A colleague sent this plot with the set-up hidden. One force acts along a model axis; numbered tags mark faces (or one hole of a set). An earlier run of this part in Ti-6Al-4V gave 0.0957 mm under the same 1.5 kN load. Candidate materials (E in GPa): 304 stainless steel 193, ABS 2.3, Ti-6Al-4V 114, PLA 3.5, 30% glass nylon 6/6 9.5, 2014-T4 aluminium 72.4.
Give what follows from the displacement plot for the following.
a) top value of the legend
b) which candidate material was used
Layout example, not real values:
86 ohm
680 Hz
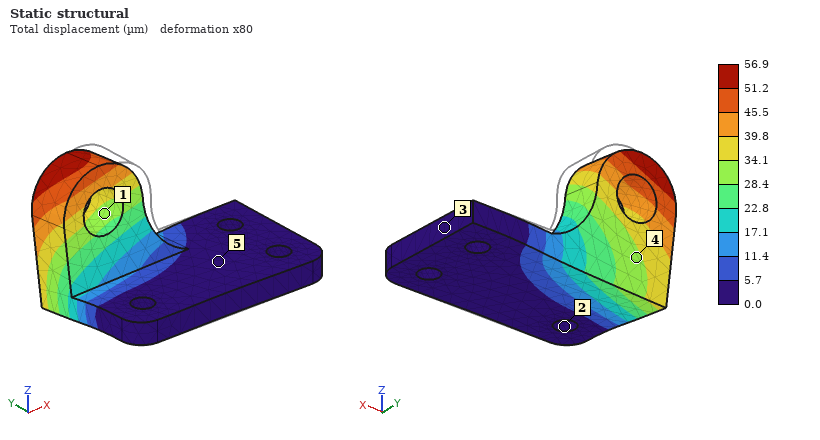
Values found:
56.9 µm
304 stainless steel
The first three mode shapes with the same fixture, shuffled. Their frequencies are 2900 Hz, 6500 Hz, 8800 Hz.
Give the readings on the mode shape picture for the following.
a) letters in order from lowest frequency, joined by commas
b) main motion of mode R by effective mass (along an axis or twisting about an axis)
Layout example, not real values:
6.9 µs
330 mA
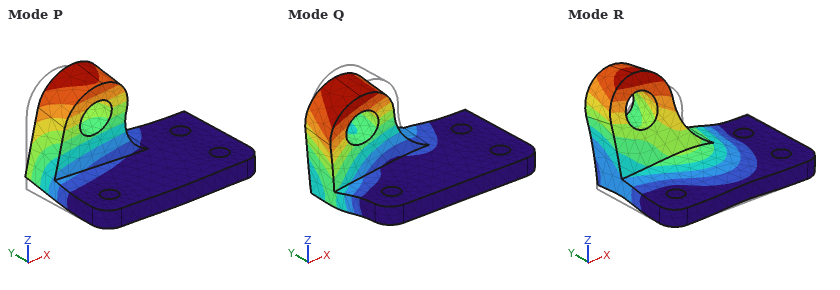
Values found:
P, Q, R
along Z
